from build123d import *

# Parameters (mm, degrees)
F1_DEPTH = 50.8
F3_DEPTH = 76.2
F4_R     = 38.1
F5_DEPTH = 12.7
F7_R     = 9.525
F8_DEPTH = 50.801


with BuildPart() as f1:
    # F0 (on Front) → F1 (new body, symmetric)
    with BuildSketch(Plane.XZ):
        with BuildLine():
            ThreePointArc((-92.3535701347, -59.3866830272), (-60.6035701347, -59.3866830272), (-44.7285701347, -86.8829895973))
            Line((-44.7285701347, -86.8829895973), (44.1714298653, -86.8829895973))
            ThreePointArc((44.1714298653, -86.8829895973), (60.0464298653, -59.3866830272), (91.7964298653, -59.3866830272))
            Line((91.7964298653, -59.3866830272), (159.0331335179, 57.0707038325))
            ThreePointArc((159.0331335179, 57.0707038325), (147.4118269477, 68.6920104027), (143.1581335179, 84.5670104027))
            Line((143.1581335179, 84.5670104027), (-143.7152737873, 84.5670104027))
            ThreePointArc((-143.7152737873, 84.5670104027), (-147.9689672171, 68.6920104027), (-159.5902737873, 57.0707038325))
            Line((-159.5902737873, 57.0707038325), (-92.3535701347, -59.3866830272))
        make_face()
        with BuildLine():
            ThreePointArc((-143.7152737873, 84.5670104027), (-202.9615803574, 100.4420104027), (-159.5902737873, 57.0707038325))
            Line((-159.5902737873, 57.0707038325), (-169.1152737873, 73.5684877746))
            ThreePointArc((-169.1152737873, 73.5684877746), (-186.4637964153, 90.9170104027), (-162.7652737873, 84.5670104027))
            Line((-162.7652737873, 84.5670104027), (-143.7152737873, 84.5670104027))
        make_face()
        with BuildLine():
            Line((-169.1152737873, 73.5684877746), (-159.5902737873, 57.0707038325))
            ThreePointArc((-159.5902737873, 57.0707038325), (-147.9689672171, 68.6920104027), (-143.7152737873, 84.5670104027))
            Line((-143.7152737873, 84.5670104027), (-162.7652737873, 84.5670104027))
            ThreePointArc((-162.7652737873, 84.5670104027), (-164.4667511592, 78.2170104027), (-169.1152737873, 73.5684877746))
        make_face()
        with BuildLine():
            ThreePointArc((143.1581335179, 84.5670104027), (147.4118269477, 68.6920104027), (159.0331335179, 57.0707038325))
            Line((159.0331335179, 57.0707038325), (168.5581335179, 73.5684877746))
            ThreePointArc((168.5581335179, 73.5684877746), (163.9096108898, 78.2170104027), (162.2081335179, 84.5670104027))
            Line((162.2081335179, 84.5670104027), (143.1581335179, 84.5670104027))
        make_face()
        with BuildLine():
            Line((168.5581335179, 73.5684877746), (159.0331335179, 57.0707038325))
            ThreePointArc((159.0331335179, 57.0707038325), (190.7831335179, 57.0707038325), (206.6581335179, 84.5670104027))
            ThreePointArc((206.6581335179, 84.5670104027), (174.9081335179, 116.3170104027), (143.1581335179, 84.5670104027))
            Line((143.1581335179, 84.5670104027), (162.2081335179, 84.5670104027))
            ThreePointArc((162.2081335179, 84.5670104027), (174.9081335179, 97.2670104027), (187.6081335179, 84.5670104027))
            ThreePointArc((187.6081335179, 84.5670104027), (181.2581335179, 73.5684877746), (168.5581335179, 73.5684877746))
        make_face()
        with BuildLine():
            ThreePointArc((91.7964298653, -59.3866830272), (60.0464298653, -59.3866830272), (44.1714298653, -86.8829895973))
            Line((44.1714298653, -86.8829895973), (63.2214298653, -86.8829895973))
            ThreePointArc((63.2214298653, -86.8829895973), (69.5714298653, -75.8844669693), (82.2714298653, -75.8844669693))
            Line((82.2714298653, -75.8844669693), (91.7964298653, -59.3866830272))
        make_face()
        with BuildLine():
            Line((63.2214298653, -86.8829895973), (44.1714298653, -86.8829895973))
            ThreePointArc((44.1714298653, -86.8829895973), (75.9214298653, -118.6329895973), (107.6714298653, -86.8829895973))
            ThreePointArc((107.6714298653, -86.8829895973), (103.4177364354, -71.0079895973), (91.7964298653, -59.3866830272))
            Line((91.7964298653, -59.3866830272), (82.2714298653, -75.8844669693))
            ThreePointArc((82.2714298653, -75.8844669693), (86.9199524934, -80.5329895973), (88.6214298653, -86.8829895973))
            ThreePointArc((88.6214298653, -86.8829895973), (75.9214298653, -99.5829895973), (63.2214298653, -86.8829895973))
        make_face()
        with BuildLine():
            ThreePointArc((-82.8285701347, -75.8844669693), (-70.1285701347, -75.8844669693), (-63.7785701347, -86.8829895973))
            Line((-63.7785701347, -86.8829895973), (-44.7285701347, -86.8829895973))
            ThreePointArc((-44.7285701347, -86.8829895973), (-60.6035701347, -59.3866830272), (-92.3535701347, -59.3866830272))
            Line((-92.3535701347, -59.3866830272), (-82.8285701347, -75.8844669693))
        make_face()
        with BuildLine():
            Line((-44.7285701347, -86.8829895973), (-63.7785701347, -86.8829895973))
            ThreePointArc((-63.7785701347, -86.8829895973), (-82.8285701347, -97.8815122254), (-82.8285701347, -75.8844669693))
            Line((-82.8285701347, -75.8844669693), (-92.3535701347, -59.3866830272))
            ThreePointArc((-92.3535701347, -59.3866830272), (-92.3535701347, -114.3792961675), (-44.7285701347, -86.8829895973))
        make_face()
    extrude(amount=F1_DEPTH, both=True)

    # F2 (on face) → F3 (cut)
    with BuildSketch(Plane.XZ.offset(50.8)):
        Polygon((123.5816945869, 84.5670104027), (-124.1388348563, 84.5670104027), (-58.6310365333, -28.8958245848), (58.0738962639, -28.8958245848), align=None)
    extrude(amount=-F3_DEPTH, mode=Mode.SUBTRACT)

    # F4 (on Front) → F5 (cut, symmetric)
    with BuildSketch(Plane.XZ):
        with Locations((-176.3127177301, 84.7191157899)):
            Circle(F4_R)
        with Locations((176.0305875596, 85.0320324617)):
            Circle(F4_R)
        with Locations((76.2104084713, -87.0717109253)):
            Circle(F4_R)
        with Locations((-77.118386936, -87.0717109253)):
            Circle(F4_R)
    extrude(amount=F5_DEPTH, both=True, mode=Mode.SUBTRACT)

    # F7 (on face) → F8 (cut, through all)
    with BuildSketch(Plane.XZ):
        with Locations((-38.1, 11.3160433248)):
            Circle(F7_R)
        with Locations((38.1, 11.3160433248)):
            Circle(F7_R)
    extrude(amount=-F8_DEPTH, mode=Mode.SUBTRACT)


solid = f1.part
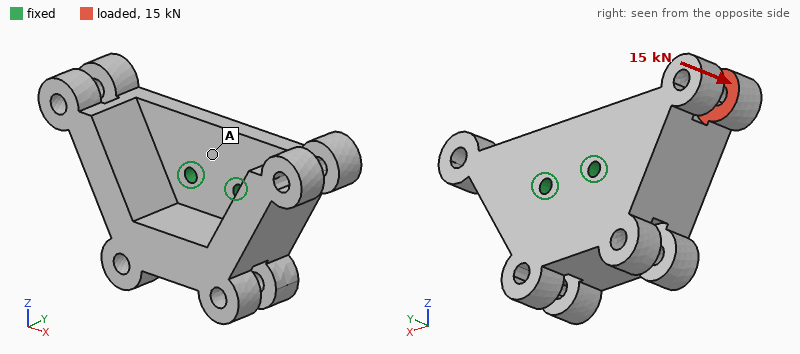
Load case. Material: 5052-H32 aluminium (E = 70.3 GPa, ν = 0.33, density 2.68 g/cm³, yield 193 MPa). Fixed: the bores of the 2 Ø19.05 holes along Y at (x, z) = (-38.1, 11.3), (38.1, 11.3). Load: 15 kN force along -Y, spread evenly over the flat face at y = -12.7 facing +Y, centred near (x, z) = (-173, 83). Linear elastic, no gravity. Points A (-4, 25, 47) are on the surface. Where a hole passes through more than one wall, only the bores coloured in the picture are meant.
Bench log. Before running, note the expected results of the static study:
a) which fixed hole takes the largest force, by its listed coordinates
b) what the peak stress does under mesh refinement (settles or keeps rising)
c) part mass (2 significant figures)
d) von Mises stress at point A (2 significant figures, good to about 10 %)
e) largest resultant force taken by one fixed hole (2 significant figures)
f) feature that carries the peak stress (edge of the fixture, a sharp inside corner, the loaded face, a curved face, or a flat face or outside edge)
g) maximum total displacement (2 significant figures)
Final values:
(-38.1, 11.3)
keeps rising
8.7 kg
16 MPa
31 kN
edge of the fixture
0.66 mm
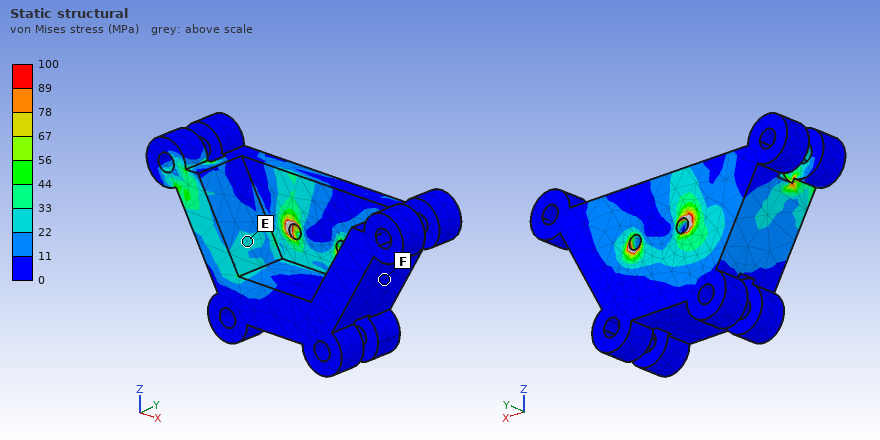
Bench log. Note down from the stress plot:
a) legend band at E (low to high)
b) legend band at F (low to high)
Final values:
22 to 33 MPa
0 to 11 MPa
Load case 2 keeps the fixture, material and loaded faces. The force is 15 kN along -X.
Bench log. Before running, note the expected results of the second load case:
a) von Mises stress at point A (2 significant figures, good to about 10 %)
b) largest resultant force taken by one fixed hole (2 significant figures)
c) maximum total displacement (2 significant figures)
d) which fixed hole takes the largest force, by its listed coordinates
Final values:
7.9 MPa
16 kN
0.35 mm
(-38.1, 11.3)
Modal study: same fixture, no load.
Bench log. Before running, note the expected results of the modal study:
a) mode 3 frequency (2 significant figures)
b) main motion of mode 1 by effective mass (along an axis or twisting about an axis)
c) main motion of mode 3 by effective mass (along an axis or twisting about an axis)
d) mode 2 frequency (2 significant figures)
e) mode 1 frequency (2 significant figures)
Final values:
1200 Hz
along Z
twisting about Y
800 Hz
650 Hz
